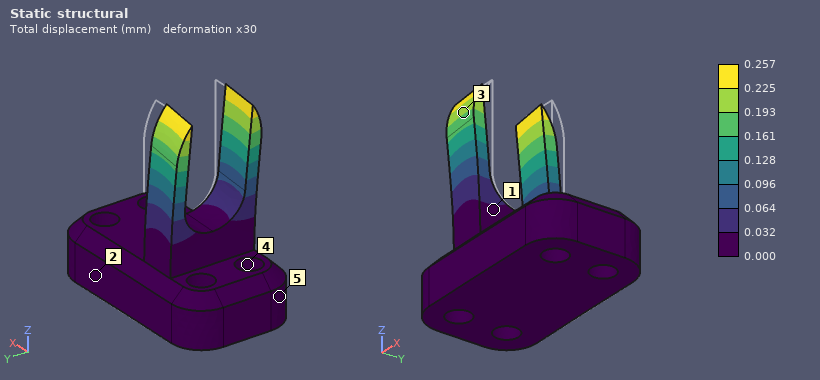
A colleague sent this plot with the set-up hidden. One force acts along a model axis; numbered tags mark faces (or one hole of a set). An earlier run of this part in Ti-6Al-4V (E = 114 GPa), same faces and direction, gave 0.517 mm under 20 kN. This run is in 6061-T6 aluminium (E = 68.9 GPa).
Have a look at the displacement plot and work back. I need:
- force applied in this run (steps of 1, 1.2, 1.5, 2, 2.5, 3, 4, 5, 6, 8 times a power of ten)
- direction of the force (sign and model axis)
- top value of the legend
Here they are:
6 kN
-X
0.257 mm
